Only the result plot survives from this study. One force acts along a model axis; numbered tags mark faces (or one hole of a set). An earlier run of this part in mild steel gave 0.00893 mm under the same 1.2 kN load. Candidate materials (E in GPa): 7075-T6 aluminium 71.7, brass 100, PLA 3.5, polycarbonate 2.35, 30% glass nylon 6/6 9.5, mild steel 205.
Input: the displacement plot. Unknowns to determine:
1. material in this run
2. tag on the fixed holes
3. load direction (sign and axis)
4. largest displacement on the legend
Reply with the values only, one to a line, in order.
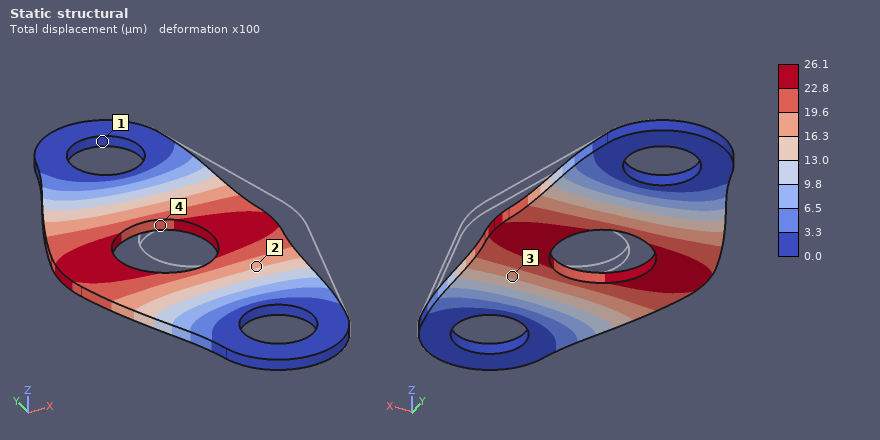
7075-T6 aluminium
1
-X
26.1 µm
